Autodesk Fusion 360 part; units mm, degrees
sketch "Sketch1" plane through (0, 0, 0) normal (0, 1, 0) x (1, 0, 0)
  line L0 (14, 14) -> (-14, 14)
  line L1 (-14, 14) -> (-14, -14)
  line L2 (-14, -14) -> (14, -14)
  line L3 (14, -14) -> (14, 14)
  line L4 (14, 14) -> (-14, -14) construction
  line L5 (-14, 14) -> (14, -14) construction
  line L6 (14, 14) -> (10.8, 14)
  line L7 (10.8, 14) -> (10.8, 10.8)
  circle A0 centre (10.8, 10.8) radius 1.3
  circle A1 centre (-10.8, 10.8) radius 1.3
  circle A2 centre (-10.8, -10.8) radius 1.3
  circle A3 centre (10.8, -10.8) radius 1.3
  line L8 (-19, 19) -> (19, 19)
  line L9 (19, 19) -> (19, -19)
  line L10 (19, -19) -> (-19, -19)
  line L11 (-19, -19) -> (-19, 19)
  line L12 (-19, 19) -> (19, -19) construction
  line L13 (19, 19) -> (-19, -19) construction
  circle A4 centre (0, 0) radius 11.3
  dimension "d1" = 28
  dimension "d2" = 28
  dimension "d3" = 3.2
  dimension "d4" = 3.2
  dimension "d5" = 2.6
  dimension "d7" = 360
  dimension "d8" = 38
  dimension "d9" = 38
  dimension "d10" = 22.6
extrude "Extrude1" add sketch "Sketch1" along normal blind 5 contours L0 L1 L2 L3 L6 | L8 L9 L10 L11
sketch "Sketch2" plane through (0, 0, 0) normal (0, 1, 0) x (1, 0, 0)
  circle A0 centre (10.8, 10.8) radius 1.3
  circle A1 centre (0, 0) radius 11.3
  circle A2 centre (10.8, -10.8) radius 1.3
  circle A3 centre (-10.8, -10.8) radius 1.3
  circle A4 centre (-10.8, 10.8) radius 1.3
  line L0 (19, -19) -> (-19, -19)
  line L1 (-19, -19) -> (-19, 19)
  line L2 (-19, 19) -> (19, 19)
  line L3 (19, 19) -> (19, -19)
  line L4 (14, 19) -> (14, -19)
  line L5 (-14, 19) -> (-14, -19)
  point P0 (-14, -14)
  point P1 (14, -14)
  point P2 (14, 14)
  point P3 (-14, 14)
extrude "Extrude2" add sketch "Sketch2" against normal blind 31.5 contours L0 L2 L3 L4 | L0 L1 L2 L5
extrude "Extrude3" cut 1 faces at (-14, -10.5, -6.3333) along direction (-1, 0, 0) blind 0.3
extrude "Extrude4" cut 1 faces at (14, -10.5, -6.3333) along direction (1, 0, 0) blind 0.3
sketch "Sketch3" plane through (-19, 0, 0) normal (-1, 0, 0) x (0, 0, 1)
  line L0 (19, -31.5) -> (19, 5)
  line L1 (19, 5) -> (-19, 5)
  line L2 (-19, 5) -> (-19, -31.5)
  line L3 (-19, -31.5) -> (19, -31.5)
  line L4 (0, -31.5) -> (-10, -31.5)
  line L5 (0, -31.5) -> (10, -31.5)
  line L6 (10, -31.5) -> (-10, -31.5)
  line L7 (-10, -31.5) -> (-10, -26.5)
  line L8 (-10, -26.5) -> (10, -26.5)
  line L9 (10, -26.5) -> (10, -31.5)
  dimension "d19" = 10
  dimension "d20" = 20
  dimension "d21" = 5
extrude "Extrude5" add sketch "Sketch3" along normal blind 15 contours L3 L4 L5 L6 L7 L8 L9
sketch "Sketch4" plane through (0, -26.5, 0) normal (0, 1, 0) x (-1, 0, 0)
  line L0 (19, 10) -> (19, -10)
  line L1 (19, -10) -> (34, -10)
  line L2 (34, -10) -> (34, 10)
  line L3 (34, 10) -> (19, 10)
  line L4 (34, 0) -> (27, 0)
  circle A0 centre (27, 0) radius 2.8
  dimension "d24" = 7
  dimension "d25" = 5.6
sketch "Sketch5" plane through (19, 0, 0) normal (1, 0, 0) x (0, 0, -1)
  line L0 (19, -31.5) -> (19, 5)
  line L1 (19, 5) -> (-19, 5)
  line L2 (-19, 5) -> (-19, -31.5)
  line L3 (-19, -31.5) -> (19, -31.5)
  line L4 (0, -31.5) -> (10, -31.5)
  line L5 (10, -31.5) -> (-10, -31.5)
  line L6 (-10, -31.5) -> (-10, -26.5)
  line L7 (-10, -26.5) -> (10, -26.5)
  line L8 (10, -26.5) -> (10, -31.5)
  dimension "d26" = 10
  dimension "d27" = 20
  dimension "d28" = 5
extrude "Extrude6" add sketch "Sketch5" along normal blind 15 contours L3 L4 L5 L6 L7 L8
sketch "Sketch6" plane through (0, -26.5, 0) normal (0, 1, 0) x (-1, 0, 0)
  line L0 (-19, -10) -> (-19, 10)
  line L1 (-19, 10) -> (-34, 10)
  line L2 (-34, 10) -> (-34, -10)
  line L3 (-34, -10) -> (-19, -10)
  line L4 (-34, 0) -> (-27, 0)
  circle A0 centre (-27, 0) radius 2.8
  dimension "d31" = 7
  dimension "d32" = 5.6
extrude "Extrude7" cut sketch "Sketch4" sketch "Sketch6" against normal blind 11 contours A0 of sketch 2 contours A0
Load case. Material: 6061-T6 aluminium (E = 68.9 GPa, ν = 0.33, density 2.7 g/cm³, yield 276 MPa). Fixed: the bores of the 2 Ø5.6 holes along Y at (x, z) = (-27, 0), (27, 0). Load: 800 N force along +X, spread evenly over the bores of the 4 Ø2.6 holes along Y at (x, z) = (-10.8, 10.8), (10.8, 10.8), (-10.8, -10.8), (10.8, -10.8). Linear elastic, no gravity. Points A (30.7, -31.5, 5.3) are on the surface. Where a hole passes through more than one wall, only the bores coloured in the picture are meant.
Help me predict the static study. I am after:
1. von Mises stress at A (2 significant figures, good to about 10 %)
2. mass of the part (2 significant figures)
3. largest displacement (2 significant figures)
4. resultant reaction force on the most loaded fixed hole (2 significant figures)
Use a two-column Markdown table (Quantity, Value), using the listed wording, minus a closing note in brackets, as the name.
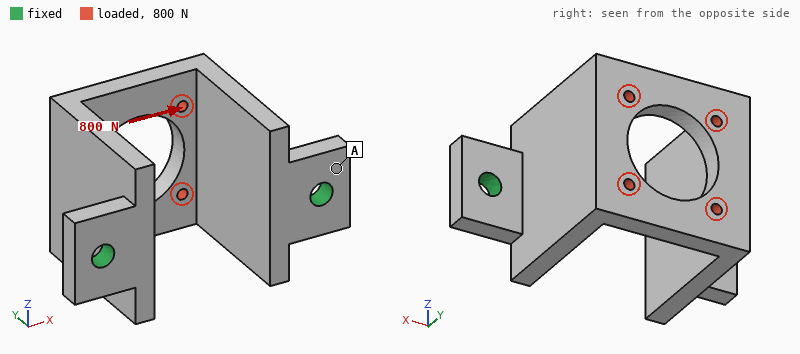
| Quantity | Value |
|---|---|
| von Mises stress at A | 6.7 MPa |
| mass of the part | 52 g |
| largest displacement | 0.11 mm |
| resultant reaction force on the most loaded fixed hole | 570 N |
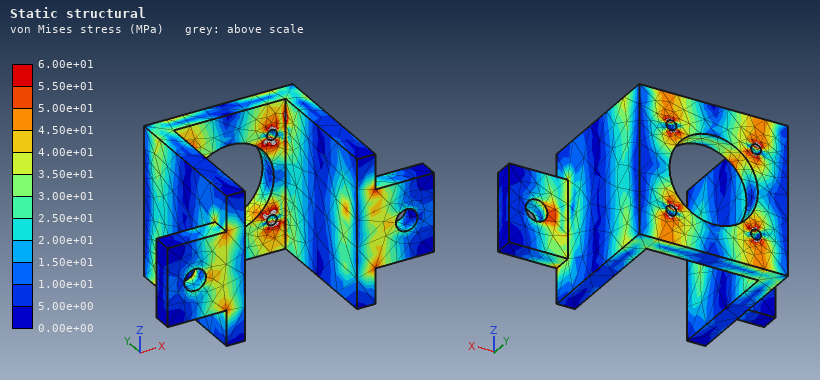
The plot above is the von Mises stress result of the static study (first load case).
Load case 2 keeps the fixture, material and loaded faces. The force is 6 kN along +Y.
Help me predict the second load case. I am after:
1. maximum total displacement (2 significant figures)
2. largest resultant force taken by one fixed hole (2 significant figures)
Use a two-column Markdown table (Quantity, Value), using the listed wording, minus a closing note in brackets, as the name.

| Quantity | Value |
|---|---|
| maximum total displacement | 91 µm |
| largest resultant force taken by one fixed hole | 3.1 kN |
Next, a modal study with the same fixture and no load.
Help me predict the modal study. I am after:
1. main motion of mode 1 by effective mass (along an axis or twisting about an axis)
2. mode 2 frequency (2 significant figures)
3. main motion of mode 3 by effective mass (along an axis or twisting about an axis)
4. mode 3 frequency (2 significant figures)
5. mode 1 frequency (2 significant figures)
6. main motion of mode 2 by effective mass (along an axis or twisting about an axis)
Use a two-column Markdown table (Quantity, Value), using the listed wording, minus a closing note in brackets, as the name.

| Quantity | Value |
|---|---|
| main motion of mode 1 by effective mass | along Z |
| mode 2 frequency | 2900 Hz |
| main motion of mode 3 by effective mass | twisting about Y |
| mode 3 frequency | 3800 Hz |
| mode 1 frequency | 2200 Hz |
| main motion of mode 2 by effective mass | along X |
